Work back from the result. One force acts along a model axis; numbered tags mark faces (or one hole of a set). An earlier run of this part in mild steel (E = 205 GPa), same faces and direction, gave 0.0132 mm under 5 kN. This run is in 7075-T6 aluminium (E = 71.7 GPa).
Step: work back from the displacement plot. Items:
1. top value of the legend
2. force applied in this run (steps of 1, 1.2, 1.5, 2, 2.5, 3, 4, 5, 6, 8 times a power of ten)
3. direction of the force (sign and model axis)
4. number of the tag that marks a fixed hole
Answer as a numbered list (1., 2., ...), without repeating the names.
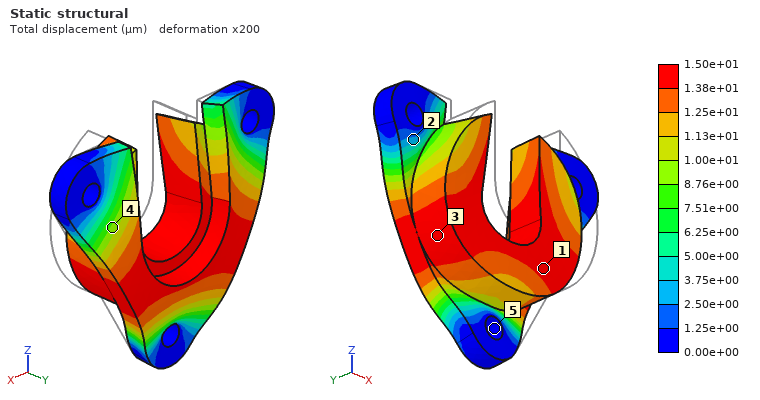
1. 1.50e+01 µm
2. 2 kN
3. +Y
4. 5
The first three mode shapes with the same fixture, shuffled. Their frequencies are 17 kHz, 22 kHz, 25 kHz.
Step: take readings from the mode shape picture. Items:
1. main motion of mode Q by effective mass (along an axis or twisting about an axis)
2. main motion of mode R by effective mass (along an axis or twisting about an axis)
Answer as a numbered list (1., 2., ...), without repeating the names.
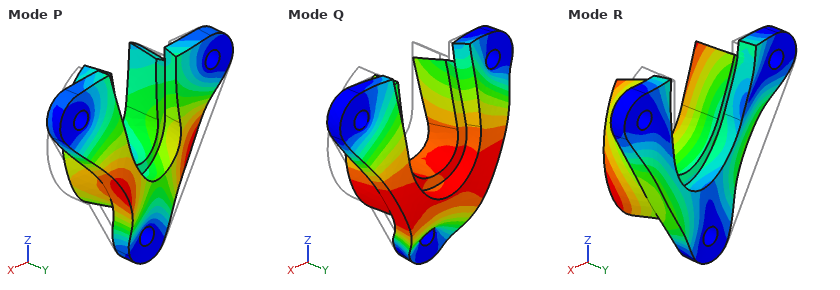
1. along Y
2. along X
